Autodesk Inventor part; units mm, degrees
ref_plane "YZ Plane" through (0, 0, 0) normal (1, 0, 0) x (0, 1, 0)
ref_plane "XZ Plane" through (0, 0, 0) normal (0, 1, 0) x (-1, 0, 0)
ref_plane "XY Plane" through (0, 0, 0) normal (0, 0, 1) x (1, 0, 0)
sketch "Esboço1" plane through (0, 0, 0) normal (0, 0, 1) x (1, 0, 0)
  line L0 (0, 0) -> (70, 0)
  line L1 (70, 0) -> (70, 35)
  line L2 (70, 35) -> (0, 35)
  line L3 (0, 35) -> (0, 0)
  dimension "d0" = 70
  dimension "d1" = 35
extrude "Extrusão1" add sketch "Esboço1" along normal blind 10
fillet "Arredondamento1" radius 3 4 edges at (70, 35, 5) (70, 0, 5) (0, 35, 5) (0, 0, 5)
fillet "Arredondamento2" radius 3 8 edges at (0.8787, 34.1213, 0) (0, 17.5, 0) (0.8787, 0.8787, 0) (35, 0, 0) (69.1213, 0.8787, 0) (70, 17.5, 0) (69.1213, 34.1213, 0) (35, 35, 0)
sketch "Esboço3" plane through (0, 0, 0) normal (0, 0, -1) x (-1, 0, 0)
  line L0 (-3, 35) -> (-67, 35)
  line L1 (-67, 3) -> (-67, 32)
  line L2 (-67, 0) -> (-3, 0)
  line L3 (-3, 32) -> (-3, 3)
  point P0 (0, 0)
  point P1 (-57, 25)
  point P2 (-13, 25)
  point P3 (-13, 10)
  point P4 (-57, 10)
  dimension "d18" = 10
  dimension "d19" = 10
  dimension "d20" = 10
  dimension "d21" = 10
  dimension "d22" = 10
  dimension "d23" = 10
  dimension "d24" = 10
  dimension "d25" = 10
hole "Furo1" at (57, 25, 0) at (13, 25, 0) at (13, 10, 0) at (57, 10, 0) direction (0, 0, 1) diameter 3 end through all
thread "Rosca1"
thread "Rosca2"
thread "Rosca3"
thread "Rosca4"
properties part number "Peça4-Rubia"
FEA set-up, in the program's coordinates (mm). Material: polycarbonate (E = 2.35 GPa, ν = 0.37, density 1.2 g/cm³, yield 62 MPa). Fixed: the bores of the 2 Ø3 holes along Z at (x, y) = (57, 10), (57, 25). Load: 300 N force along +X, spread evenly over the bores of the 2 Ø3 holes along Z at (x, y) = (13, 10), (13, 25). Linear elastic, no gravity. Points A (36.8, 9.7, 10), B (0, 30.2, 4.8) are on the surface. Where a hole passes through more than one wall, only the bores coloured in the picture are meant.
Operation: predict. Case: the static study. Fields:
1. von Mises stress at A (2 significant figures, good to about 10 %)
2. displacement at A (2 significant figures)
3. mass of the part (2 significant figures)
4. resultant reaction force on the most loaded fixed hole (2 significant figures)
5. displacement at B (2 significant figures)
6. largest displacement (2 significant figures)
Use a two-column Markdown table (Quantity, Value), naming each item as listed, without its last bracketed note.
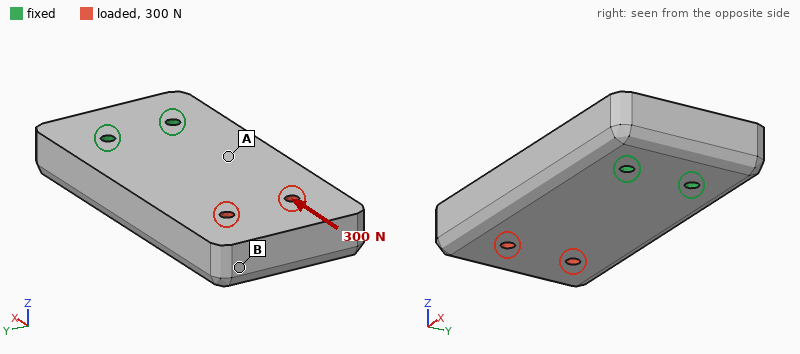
| Quantity | Value |
|---|---|
| von Mises stress at A | 0.90 MPa |
| displacement at A | 9.0 µm |
| mass of the part | 29 g |
| resultant reaction force on the most loaded fixed hole | 150 N |
| displacement at B | 18 µm |
| largest displacement | 21 µm |
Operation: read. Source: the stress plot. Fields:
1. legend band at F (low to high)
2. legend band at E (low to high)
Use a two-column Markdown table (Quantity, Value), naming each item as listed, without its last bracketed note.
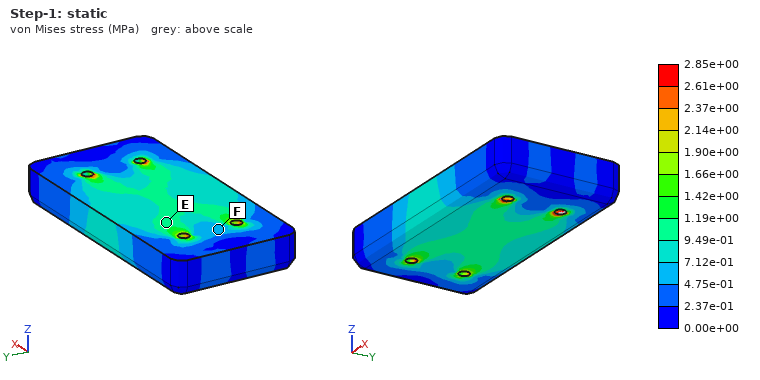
| Quantity | Value |
|---|---|
| legend band at F | 4.75e-01 to 7.12e-01 MPa |
| legend band at E | 9.49e-01 to 1.19e+00 MPa |
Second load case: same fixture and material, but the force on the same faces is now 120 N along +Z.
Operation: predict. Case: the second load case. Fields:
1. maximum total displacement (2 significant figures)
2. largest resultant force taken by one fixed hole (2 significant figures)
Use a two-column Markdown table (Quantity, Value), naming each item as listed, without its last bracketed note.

| Quantity | Value |
|---|---|
| maximum total displacement | 0.83 mm |
| largest resultant force taken by one fixed hole | 60 N |
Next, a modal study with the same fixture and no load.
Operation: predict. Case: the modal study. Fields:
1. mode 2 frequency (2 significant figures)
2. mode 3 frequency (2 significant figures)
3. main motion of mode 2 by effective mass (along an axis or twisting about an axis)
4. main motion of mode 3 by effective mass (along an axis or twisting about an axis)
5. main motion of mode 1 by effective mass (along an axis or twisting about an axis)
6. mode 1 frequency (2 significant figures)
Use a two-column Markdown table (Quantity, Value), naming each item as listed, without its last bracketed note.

| Quantity | Value |
|---|---|
| mode 2 frequency | 1500 Hz |
| mode 3 frequency | 2000 Hz |
| main motion of mode 2 by effective mass | along Y |
| main motion of mode 3 by effective mass | twisting about X |
| main motion of mode 1 by effective mass | along Z |
| mode 1 frequency | 650 Hz |
